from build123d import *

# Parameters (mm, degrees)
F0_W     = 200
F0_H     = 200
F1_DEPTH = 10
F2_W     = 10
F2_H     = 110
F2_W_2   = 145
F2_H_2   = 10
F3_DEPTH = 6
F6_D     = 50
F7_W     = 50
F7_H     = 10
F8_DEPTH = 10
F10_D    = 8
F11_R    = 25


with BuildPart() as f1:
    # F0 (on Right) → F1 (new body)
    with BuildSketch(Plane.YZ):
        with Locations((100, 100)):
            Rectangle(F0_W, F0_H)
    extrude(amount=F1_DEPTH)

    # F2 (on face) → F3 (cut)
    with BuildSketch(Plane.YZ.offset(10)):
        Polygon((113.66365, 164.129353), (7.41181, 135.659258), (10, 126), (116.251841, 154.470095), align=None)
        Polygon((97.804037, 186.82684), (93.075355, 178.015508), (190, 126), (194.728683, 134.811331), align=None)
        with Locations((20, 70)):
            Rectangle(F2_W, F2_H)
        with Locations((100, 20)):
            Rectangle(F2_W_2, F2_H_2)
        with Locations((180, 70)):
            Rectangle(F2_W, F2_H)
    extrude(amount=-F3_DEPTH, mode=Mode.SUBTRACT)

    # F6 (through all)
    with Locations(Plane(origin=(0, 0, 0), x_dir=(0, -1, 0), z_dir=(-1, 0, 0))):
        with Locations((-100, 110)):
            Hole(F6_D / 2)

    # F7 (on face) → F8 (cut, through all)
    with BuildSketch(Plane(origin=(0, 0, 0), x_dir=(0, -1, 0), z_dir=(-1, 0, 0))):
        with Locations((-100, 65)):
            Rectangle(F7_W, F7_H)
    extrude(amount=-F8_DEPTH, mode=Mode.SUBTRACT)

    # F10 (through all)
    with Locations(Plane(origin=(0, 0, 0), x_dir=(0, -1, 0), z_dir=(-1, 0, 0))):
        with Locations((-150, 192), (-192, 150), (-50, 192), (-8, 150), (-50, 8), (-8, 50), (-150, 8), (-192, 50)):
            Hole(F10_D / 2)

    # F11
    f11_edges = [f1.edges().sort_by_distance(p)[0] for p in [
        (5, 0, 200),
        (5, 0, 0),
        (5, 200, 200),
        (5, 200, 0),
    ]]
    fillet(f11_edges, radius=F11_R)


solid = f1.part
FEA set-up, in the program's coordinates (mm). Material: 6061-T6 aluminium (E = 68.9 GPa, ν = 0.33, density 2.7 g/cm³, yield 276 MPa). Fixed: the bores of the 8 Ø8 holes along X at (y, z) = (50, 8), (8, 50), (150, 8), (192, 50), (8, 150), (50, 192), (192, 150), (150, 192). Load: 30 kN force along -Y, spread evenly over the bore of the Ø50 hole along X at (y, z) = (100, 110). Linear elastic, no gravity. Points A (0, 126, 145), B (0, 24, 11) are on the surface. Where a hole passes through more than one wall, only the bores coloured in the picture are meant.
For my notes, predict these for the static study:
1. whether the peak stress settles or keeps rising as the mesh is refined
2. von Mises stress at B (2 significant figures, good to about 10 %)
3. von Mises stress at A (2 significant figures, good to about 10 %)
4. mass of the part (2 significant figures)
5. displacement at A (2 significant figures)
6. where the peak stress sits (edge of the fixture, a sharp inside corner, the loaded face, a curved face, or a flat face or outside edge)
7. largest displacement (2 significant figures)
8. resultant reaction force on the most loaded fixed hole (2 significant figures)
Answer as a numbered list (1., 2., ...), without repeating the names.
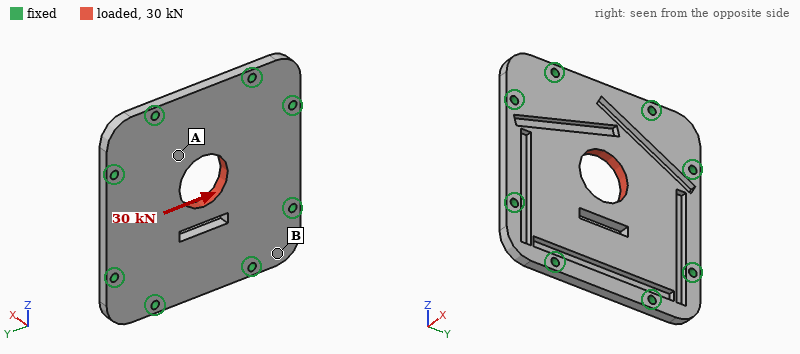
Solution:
1. keeps rising
2. 7.0 MPa
3. 23 MPa
4. 890 g
5. 19 µm
6. edge of the fixture
7. 35 µm
8. 6.2 kN
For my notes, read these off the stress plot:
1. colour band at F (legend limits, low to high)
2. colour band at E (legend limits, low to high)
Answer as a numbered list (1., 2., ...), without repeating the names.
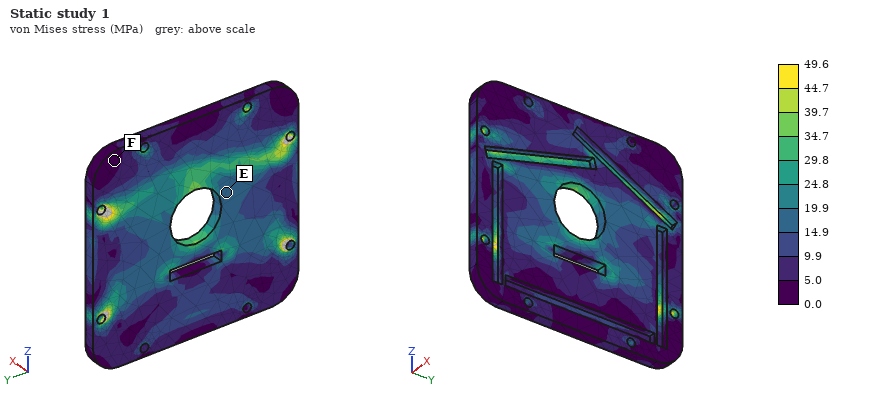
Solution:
1. 0.0 to 5.0 MPa
2. 14.9 to 19.9 MPa
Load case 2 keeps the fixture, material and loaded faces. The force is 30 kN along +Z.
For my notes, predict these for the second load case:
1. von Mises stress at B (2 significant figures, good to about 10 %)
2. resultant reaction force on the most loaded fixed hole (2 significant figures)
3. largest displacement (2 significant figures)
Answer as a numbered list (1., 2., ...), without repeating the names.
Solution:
1. 9.7 MPa
2. 5.9 kN
3. 56 µm
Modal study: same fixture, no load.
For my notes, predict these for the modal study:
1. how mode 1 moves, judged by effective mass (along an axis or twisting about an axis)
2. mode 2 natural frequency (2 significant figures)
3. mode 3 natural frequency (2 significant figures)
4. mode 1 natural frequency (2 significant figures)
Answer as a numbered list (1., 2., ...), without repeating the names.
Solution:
1. along X
2. 3200 Hz
3. 3200 Hz
4. 1600 Hz
